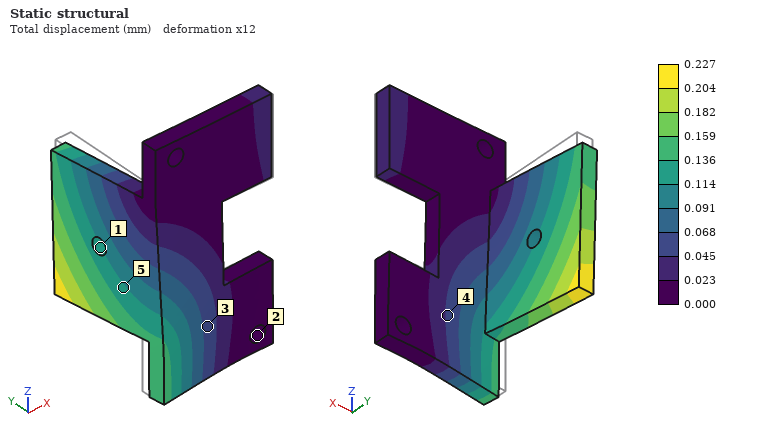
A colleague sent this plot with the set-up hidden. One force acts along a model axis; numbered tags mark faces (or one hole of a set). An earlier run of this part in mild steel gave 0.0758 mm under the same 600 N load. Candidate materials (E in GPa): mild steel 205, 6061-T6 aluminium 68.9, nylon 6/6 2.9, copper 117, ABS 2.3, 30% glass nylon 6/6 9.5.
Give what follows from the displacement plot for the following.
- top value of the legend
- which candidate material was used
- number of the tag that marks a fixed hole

0.227 mm
6061-T6 aluminium
2
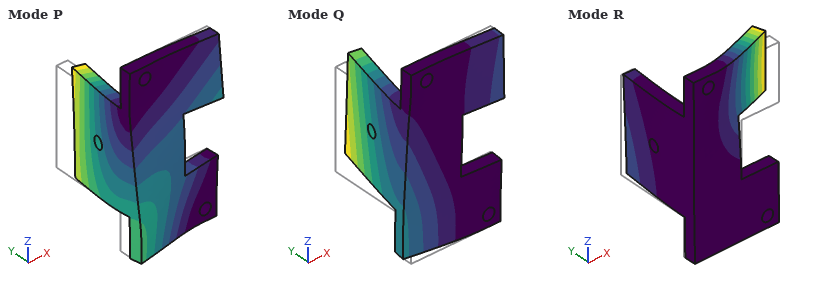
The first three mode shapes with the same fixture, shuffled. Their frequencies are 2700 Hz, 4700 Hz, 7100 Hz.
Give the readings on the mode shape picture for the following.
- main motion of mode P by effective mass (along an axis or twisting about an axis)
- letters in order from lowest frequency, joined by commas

along Y
Q, P, R
